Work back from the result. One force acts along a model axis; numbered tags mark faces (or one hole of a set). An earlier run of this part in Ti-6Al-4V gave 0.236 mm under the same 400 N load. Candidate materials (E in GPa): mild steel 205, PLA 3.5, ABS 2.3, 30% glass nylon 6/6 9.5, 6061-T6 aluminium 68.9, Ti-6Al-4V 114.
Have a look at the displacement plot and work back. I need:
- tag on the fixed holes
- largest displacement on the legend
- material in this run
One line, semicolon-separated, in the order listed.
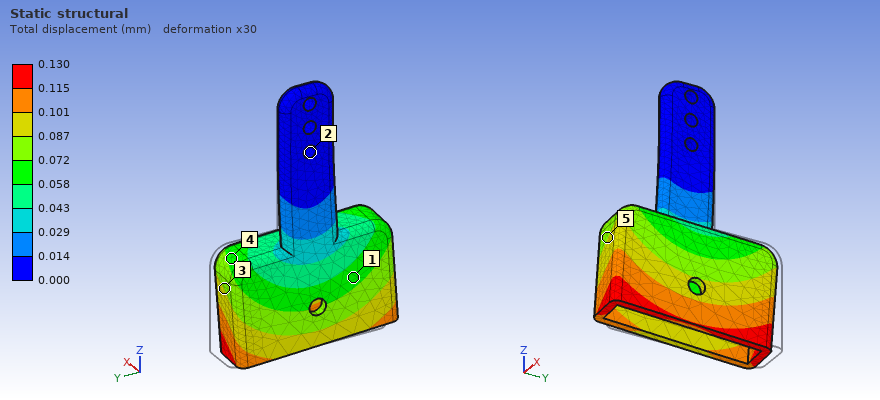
2; 0.130 mm; mild steel
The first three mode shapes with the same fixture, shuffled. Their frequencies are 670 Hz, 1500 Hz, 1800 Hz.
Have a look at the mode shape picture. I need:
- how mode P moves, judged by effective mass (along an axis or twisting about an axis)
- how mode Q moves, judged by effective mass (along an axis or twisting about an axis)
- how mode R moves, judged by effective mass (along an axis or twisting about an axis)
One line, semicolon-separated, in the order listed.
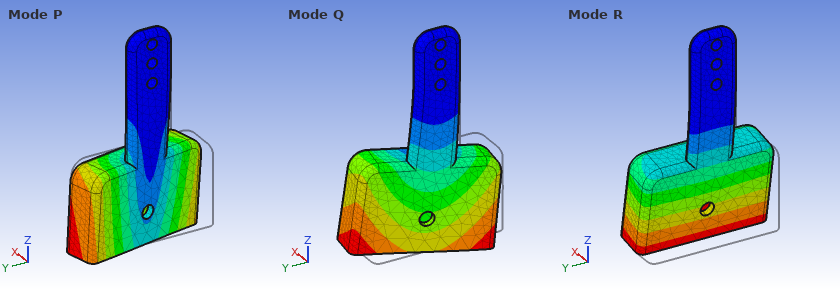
along Y; along Y; along X
